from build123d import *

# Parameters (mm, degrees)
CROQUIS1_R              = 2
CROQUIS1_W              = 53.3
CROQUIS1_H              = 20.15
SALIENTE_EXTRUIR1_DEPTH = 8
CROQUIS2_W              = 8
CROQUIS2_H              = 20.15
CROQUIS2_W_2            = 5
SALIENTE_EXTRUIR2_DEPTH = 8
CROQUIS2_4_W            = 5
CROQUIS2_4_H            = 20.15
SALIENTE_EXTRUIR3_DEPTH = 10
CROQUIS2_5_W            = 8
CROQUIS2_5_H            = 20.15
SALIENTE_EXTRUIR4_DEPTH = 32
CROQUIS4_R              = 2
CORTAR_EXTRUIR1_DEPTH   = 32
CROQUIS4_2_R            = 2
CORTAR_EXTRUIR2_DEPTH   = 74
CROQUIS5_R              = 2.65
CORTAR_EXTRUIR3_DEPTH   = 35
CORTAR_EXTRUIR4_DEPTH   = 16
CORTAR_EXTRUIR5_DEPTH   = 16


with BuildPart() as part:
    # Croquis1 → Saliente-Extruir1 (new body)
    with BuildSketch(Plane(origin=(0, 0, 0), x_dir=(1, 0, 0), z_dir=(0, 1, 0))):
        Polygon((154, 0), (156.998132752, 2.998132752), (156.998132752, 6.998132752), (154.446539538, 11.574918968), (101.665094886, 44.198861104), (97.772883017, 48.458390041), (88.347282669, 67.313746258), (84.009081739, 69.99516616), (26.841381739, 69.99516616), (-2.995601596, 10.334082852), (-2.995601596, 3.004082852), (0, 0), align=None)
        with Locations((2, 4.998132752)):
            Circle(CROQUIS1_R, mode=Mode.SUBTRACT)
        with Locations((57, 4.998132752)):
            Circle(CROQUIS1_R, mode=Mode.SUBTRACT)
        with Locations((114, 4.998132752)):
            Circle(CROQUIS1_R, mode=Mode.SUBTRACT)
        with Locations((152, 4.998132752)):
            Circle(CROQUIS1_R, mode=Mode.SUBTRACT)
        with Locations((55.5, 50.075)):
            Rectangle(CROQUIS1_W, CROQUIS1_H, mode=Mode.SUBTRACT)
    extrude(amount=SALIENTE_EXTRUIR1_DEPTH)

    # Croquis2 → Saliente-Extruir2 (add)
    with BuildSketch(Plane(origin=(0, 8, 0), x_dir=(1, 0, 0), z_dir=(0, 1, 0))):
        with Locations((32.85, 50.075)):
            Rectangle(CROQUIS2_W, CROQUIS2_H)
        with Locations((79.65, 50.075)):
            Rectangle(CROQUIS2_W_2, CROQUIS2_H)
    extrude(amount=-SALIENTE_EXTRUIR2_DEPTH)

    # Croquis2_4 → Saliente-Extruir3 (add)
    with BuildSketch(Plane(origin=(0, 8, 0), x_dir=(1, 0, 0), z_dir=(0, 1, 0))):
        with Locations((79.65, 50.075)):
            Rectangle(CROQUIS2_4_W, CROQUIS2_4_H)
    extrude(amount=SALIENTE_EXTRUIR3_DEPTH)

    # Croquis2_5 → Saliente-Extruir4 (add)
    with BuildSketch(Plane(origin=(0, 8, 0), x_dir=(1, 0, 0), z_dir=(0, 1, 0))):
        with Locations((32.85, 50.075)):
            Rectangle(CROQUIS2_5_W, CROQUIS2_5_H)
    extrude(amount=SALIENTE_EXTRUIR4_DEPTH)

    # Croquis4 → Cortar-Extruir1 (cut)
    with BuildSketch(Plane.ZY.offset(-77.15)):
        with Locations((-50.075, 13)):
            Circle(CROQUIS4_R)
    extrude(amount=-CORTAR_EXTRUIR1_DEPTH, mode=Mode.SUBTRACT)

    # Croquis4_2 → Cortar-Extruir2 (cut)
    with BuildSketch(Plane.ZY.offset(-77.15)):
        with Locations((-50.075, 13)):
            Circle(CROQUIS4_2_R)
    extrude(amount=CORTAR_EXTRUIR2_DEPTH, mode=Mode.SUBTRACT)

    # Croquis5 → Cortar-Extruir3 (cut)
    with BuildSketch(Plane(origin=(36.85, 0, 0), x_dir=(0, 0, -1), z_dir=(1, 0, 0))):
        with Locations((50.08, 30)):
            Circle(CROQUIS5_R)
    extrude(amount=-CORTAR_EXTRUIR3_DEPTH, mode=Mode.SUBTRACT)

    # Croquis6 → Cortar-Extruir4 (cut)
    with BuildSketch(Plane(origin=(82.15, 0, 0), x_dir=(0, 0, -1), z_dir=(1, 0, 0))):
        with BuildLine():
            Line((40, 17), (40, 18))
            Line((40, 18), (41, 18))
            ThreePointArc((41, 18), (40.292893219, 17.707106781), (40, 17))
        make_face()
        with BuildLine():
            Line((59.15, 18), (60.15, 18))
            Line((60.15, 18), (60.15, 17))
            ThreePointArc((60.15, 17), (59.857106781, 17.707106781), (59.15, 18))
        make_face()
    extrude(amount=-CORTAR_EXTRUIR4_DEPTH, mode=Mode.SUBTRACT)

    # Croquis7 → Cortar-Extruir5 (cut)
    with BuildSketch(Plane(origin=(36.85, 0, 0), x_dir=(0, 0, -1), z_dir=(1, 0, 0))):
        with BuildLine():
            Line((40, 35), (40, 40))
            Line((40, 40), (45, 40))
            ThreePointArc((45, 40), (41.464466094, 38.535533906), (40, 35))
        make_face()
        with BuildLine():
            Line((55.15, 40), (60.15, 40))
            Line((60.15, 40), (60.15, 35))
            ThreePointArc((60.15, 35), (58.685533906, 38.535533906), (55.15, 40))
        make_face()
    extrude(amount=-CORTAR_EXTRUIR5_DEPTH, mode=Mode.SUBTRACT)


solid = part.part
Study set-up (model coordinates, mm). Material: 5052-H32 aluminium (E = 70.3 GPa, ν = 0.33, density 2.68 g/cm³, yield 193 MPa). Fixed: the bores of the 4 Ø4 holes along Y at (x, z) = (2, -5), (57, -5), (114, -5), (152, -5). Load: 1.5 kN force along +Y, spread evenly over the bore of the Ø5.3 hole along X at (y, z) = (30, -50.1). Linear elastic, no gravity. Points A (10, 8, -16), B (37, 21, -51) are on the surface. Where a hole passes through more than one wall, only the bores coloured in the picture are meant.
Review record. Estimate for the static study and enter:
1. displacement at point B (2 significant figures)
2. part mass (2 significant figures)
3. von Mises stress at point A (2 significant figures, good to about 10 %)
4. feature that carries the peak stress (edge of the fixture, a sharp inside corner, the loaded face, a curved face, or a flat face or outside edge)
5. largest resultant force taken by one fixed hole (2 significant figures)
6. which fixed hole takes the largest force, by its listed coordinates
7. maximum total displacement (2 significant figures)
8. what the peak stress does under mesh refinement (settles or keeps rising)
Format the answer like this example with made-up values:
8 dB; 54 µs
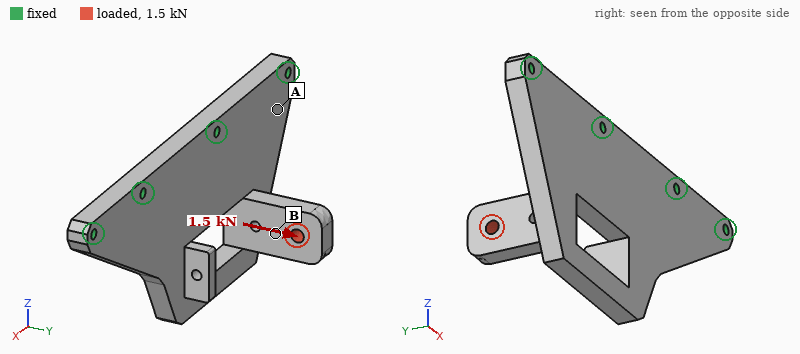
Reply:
0.38 mm; 160 g; 70 MPa; edge of the fixture; 1.0 kN; (57, -5); 0.55 mm; keeps rising
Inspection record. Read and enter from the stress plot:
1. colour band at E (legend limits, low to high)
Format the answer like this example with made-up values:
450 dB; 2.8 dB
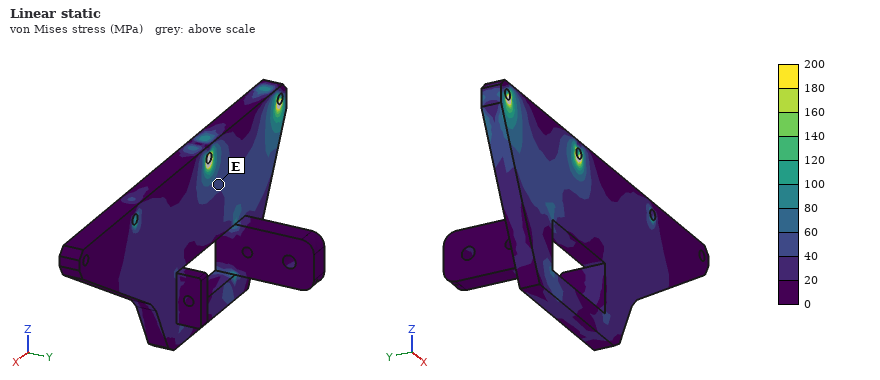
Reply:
40 to 60 MPa
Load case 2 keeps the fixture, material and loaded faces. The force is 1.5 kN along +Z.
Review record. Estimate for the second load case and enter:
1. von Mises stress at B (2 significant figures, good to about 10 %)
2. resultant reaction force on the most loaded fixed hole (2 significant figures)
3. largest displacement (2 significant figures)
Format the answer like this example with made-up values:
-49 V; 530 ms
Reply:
28 MPa; 840 N; 0.57 mm
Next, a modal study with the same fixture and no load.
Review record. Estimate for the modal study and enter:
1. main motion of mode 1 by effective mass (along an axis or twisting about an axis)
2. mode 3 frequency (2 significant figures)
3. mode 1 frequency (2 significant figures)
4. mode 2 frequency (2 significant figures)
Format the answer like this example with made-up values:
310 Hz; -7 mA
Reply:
along Y; 4000 Hz; 1400 Hz; 2800 Hz
